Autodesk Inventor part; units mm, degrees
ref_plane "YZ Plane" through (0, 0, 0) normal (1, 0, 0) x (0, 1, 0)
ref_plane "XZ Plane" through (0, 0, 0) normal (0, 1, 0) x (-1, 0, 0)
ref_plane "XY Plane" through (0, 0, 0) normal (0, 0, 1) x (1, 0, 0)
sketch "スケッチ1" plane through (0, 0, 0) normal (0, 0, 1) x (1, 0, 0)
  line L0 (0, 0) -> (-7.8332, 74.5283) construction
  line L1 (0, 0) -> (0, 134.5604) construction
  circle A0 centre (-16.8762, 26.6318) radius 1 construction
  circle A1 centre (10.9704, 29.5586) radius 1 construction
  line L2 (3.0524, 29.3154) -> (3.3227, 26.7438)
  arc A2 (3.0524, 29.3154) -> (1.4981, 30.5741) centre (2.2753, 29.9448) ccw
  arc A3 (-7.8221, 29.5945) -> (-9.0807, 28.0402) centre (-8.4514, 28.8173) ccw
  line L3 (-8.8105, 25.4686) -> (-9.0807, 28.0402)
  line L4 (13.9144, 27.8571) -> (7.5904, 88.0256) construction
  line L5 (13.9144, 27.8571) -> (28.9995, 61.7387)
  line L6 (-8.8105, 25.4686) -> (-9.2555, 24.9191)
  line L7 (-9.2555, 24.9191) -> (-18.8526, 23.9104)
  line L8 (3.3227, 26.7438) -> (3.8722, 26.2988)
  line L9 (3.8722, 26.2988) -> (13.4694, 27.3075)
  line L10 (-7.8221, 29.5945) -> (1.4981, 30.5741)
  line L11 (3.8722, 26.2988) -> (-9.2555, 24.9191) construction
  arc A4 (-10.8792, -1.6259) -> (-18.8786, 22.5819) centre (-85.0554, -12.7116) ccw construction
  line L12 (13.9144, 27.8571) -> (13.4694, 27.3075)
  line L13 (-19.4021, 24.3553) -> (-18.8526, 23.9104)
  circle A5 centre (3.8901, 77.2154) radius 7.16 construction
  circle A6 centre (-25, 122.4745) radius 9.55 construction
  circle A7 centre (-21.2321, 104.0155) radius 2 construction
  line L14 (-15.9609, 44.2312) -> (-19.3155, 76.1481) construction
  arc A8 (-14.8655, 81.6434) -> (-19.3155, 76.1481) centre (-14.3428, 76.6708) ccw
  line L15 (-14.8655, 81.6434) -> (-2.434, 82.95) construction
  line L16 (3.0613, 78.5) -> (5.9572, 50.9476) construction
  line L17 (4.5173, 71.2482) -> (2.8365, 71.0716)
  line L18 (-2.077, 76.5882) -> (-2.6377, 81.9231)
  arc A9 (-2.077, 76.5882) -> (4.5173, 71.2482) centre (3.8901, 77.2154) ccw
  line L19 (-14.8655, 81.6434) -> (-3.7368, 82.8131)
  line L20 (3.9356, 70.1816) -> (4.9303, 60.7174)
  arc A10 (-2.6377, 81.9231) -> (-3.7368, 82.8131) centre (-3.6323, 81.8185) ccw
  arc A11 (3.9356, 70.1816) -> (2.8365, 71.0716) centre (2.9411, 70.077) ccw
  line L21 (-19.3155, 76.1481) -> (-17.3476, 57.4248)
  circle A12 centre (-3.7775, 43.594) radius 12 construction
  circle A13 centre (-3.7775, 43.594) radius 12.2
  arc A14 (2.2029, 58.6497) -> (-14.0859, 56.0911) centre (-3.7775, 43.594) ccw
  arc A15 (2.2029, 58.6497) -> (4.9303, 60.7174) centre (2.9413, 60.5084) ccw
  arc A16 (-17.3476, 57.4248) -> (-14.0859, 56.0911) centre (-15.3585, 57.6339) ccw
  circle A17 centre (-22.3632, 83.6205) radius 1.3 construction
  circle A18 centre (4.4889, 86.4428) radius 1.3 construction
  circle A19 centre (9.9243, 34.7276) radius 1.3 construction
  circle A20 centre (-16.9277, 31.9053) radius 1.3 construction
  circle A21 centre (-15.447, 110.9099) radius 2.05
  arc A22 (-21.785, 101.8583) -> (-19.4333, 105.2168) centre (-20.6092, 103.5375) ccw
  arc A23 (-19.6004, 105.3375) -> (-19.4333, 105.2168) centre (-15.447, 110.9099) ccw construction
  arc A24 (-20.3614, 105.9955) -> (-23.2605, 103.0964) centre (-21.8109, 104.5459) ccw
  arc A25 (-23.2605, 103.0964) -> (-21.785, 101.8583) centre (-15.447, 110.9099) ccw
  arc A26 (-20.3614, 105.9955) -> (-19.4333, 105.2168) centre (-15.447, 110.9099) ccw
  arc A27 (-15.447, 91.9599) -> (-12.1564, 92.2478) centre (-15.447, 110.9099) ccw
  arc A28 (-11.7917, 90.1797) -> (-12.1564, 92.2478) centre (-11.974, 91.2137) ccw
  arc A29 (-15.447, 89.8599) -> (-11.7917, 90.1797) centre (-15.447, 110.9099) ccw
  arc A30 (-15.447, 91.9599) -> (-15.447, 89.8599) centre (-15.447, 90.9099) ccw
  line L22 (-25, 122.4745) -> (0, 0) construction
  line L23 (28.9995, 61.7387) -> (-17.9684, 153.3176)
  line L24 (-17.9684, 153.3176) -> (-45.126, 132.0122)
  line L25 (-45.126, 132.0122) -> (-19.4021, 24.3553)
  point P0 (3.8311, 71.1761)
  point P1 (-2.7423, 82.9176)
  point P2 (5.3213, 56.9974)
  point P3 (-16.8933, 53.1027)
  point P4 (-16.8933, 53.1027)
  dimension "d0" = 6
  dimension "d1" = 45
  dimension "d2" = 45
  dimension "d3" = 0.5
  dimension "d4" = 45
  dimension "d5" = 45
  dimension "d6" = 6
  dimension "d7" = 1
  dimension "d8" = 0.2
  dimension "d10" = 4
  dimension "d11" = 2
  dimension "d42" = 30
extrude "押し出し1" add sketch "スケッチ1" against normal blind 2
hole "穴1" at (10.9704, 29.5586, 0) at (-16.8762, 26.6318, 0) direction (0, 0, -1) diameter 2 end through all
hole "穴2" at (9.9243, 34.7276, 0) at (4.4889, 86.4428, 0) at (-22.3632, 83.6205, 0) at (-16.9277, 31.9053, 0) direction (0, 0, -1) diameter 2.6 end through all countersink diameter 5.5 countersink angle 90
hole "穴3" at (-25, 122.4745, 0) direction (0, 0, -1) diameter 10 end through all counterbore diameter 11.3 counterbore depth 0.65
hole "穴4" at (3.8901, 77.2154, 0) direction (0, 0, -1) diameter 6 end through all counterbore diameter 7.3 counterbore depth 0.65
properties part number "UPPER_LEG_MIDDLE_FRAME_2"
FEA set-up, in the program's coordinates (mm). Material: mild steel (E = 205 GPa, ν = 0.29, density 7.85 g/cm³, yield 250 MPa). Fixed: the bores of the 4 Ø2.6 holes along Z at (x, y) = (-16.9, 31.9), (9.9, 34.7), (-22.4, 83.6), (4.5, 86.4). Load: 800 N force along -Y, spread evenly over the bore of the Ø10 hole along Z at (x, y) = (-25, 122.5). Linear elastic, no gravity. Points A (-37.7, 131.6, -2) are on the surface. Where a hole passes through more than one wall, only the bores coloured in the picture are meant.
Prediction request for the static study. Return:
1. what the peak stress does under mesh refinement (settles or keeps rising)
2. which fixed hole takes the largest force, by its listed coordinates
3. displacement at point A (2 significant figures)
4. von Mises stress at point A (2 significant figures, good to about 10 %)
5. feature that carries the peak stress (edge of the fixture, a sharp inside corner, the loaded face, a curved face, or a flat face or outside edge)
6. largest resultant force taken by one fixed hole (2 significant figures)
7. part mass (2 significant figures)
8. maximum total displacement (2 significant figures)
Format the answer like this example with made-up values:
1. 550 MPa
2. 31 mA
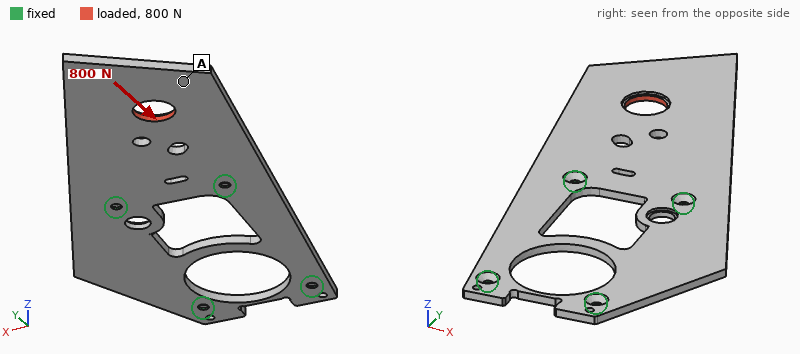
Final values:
1. keeps rising
2. (-22.4, 83.6)
3. 34 µm
4. 6.0 MPa
5. edge of the fixture
6. 670 N
7. 66 g
8. 66 µm
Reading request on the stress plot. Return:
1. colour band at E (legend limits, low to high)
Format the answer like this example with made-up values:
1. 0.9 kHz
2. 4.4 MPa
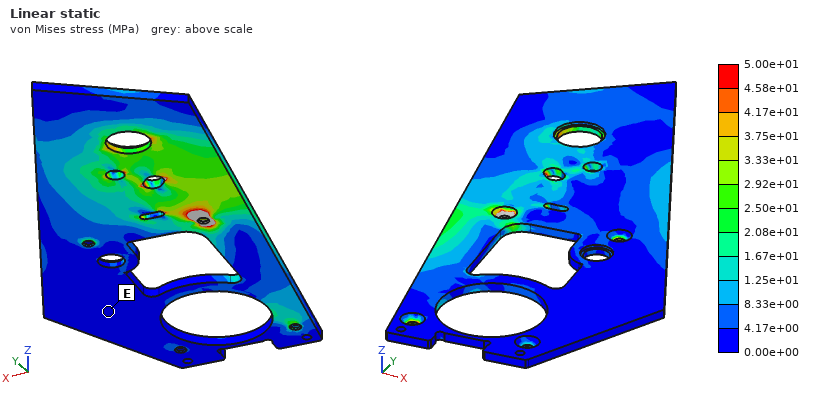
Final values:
1. 0.00e+00 to 4.17e+00 MPa
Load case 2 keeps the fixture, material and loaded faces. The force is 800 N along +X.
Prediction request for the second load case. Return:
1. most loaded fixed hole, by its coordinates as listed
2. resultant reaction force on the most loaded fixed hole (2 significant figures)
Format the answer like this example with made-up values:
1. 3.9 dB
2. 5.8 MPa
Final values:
1. (4.5, 86.4)
2. 910 N
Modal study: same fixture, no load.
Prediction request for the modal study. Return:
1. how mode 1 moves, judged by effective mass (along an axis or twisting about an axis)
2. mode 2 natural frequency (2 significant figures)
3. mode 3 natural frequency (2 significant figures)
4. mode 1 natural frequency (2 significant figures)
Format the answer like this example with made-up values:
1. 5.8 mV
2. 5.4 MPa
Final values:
1. along Z
2. 1600 Hz
3. 2100 Hz
4. 410 Hz
